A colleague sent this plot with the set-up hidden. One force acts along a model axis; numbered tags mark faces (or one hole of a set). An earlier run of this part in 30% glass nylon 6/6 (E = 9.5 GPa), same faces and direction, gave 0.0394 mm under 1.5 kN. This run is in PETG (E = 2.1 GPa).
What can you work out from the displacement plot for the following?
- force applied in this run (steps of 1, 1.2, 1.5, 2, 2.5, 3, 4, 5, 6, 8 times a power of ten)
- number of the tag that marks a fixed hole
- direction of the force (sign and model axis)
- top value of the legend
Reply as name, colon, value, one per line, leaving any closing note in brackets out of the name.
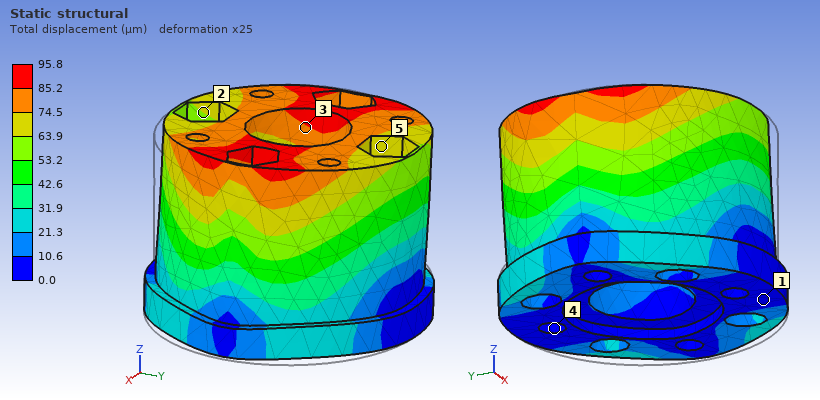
force applied in this run: 800 N
number of the tag that marks a fixed hole: 4
direction of the force: -X
top value of the legend: 95.8 µm
